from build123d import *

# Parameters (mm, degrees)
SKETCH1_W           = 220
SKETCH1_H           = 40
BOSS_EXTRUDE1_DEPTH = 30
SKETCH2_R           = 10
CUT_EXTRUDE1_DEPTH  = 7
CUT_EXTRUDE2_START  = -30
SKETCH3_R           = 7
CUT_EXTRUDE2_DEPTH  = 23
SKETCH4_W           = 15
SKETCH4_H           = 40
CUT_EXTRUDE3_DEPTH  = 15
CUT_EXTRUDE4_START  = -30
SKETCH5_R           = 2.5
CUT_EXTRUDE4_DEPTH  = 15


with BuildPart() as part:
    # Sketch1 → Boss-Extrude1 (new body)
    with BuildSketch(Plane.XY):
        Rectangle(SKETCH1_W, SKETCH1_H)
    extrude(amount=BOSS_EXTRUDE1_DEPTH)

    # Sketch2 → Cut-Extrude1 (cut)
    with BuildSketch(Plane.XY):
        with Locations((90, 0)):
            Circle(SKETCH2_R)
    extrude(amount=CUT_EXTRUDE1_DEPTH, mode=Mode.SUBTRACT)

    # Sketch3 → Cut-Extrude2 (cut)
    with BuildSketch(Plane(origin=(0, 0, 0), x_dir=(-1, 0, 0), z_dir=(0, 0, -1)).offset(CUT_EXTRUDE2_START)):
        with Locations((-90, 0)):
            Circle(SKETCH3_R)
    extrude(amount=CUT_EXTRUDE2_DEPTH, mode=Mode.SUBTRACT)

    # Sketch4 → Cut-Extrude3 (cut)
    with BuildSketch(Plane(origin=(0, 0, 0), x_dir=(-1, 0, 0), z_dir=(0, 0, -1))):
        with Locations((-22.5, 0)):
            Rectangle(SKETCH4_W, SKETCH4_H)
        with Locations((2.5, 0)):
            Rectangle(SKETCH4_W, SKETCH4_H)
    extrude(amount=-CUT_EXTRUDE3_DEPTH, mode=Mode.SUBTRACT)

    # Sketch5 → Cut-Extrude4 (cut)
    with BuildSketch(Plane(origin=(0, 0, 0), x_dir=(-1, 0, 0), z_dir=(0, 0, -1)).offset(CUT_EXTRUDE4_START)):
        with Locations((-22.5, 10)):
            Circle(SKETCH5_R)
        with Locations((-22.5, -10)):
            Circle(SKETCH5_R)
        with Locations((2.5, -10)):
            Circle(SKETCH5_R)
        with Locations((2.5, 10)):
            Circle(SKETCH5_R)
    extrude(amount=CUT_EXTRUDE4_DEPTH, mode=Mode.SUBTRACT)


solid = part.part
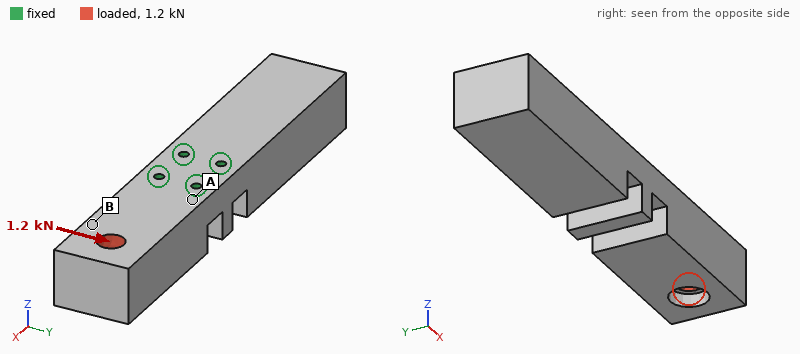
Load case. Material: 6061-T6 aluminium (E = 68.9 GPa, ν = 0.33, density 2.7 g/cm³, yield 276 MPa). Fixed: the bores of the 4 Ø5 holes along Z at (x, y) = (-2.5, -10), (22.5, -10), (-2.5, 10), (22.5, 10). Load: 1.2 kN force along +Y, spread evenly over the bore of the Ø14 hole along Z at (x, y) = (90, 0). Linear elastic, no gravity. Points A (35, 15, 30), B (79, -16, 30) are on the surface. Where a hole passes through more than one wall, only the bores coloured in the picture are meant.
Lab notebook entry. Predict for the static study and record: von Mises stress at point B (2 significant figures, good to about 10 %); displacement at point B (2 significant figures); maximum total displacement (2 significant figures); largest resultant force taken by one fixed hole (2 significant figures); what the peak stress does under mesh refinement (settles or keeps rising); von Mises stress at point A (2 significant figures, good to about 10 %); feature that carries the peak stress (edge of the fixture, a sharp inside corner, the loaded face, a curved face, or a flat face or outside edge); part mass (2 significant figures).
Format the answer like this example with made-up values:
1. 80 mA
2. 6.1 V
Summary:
1. 2.5 MPa
2. 23 µm
3. 37 µm
4. 2.8 kN
5. keeps rising
6. 9.8 MPa
7. edge of the fixture
8. 650 g
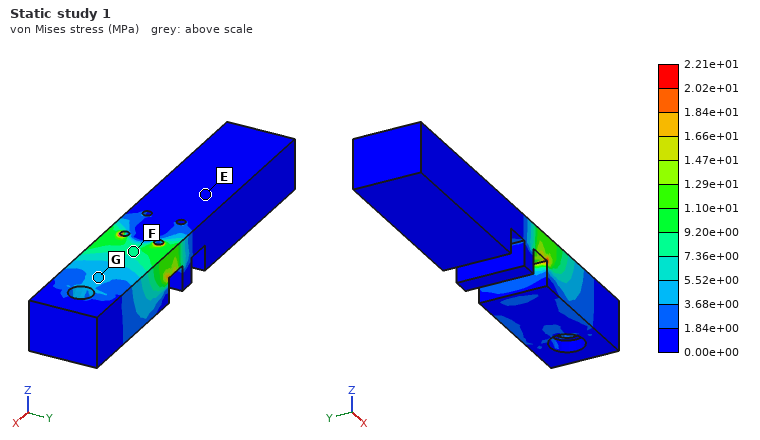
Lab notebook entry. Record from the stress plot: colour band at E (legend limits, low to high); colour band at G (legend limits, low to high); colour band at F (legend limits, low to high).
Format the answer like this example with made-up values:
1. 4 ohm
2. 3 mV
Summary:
1. 0.00e+00 to 1.84e+00 MPa
2. 3.68e+00 to 5.52e+00 MPa
3. 7.36e+00 to 9.20e+00 MPa
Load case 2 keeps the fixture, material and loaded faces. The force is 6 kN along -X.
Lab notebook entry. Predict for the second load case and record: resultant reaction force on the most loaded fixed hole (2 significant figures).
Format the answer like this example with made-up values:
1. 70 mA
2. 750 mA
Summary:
1. 2.7 kN
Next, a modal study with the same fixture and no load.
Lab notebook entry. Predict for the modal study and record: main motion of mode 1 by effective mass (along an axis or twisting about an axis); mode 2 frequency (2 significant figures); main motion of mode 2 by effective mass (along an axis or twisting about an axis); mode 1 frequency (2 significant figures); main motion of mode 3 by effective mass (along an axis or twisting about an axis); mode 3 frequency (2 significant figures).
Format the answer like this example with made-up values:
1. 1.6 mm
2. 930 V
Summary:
1. along Z
2. 1500 Hz
3. along Z
4. 990 Hz
5. along Y
6. 1900 Hz
